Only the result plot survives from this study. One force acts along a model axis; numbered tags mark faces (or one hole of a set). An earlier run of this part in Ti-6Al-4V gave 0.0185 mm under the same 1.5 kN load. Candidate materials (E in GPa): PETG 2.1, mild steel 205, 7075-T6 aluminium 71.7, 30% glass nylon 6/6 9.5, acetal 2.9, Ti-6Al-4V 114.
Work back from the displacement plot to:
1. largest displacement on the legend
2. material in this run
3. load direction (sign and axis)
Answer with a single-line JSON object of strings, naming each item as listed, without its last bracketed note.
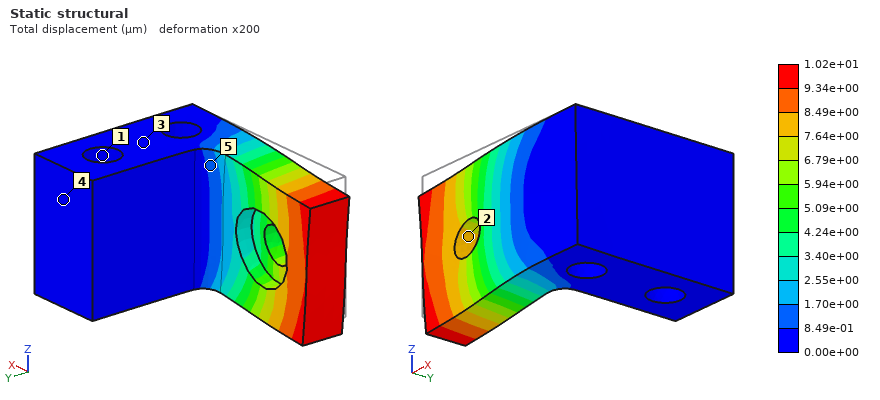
{"largest displacement on the legend": "1.02e+01 µm", "material in this run": "mild steel", "load direction": "-Z"}
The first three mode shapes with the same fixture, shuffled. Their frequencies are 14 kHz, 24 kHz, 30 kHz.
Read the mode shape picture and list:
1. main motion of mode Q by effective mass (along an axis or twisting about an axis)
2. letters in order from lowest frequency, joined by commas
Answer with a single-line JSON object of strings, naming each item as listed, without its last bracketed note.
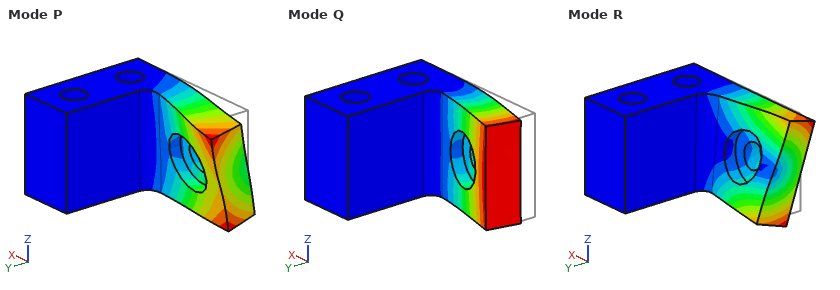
{"main motion of mode Q by effective mass": "along Y", "letters in order from lowest frequency, joined by commas": "Q, P, R"}
